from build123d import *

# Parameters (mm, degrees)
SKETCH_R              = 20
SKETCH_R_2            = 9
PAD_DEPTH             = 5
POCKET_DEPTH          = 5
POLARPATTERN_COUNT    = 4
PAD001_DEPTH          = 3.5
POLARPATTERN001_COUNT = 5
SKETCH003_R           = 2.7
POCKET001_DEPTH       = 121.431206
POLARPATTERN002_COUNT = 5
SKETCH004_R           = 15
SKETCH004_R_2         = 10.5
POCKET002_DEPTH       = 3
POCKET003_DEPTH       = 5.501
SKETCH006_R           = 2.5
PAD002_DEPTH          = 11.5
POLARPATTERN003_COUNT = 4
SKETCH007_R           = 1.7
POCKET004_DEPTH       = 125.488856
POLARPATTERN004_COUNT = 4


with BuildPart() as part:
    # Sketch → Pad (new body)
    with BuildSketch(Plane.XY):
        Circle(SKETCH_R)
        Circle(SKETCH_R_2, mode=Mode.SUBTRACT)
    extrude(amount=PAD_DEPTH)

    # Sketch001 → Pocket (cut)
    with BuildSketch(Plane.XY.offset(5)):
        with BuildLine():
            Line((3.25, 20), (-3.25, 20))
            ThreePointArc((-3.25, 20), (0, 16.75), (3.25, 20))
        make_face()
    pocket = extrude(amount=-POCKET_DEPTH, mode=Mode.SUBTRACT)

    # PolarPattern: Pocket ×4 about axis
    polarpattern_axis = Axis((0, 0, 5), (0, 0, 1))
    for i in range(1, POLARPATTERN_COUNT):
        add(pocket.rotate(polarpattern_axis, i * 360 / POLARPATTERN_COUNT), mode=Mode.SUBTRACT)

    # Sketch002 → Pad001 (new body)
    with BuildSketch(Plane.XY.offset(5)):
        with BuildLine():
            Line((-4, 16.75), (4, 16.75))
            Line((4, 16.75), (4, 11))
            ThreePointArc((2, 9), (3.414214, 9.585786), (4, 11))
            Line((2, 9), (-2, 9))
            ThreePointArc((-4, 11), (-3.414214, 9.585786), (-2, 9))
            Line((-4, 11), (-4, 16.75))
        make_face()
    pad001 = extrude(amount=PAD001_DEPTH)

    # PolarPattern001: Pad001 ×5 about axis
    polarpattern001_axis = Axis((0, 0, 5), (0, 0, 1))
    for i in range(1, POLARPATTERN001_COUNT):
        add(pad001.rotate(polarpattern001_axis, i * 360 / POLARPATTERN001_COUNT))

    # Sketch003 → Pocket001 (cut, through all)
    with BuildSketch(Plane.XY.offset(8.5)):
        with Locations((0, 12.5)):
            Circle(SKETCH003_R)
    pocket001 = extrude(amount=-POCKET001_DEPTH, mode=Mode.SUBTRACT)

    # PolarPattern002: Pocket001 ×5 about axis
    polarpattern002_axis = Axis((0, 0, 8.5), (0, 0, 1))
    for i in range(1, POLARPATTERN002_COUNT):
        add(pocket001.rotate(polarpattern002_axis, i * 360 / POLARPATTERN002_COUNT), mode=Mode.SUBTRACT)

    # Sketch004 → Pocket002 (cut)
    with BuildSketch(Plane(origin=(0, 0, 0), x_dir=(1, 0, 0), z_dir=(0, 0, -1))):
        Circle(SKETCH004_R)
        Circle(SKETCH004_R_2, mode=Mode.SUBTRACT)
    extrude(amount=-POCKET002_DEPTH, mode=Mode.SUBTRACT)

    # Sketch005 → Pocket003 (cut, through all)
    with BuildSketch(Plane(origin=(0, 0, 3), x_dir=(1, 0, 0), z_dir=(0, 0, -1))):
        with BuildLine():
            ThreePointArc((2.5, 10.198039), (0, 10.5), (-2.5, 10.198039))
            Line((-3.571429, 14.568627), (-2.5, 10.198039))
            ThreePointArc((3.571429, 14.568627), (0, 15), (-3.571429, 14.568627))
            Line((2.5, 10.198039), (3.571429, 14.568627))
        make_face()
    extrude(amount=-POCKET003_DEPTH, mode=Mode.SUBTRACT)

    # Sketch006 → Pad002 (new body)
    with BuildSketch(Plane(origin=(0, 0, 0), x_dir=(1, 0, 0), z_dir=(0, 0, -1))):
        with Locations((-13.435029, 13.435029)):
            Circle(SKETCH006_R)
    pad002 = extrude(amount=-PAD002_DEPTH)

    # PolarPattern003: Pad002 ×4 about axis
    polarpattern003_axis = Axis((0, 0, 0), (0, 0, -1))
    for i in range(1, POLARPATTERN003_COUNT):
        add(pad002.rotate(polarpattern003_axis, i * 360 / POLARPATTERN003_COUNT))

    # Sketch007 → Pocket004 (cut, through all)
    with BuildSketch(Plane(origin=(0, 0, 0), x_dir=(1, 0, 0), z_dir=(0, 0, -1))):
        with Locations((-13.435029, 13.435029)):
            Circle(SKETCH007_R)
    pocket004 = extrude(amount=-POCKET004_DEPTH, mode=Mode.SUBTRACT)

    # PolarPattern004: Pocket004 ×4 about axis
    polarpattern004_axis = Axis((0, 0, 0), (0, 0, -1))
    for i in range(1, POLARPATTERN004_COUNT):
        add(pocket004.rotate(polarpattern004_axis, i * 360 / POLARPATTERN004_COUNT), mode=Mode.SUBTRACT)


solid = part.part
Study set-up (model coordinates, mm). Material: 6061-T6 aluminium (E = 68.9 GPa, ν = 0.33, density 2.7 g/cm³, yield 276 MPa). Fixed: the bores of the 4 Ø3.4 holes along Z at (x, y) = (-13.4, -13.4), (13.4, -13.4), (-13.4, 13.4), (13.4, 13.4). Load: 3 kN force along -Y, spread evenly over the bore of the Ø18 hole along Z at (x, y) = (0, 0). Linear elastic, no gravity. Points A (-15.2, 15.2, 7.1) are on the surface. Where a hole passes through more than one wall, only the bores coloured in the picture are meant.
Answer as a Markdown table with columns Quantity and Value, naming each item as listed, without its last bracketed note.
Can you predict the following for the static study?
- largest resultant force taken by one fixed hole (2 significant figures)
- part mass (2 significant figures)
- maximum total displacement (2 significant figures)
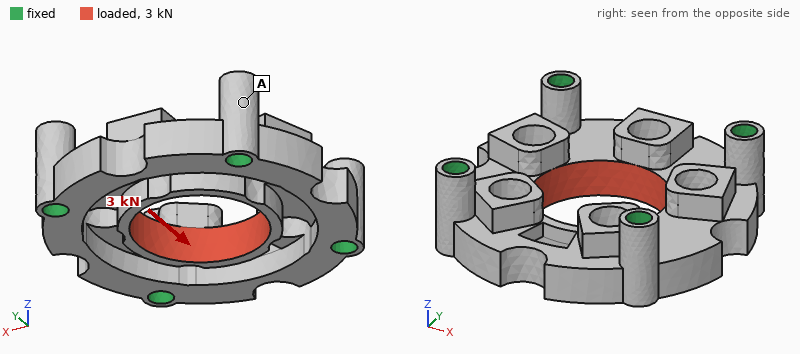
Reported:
| Quantity | Value |
|---|---|
| largest resultant force taken by one fixed hole | 850 N |
| part mass | 11 g |
| maximum total displacement | 30 µm |
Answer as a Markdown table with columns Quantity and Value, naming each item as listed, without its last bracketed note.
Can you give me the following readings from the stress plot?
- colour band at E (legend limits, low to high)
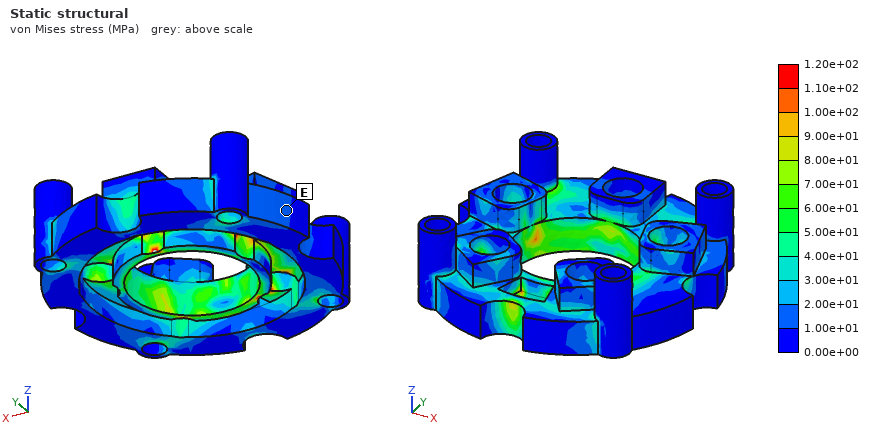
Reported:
| Quantity | Value |
|---|---|
| colour band at E | 1.00e+01 to 2.00e+01 MPa |
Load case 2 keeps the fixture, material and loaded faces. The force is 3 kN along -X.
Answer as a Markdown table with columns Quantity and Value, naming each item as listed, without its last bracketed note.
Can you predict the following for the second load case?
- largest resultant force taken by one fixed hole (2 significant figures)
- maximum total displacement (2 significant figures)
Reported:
| Quantity | Value |
|---|---|
| largest resultant force taken by one fixed hole | 790 N |
| maximum total displacement | 34 µm |
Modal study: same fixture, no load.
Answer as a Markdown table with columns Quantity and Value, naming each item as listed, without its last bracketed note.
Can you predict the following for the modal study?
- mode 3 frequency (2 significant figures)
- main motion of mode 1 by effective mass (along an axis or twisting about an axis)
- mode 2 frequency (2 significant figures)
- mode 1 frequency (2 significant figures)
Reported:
| Quantity | Value |
|---|---|
| mode 3 frequency | 29 kHz |
| main motion of mode 1 by effective mass | along Z |
| mode 2 frequency | 28 kHz |
| mode 1 frequency | 26 kHz |
